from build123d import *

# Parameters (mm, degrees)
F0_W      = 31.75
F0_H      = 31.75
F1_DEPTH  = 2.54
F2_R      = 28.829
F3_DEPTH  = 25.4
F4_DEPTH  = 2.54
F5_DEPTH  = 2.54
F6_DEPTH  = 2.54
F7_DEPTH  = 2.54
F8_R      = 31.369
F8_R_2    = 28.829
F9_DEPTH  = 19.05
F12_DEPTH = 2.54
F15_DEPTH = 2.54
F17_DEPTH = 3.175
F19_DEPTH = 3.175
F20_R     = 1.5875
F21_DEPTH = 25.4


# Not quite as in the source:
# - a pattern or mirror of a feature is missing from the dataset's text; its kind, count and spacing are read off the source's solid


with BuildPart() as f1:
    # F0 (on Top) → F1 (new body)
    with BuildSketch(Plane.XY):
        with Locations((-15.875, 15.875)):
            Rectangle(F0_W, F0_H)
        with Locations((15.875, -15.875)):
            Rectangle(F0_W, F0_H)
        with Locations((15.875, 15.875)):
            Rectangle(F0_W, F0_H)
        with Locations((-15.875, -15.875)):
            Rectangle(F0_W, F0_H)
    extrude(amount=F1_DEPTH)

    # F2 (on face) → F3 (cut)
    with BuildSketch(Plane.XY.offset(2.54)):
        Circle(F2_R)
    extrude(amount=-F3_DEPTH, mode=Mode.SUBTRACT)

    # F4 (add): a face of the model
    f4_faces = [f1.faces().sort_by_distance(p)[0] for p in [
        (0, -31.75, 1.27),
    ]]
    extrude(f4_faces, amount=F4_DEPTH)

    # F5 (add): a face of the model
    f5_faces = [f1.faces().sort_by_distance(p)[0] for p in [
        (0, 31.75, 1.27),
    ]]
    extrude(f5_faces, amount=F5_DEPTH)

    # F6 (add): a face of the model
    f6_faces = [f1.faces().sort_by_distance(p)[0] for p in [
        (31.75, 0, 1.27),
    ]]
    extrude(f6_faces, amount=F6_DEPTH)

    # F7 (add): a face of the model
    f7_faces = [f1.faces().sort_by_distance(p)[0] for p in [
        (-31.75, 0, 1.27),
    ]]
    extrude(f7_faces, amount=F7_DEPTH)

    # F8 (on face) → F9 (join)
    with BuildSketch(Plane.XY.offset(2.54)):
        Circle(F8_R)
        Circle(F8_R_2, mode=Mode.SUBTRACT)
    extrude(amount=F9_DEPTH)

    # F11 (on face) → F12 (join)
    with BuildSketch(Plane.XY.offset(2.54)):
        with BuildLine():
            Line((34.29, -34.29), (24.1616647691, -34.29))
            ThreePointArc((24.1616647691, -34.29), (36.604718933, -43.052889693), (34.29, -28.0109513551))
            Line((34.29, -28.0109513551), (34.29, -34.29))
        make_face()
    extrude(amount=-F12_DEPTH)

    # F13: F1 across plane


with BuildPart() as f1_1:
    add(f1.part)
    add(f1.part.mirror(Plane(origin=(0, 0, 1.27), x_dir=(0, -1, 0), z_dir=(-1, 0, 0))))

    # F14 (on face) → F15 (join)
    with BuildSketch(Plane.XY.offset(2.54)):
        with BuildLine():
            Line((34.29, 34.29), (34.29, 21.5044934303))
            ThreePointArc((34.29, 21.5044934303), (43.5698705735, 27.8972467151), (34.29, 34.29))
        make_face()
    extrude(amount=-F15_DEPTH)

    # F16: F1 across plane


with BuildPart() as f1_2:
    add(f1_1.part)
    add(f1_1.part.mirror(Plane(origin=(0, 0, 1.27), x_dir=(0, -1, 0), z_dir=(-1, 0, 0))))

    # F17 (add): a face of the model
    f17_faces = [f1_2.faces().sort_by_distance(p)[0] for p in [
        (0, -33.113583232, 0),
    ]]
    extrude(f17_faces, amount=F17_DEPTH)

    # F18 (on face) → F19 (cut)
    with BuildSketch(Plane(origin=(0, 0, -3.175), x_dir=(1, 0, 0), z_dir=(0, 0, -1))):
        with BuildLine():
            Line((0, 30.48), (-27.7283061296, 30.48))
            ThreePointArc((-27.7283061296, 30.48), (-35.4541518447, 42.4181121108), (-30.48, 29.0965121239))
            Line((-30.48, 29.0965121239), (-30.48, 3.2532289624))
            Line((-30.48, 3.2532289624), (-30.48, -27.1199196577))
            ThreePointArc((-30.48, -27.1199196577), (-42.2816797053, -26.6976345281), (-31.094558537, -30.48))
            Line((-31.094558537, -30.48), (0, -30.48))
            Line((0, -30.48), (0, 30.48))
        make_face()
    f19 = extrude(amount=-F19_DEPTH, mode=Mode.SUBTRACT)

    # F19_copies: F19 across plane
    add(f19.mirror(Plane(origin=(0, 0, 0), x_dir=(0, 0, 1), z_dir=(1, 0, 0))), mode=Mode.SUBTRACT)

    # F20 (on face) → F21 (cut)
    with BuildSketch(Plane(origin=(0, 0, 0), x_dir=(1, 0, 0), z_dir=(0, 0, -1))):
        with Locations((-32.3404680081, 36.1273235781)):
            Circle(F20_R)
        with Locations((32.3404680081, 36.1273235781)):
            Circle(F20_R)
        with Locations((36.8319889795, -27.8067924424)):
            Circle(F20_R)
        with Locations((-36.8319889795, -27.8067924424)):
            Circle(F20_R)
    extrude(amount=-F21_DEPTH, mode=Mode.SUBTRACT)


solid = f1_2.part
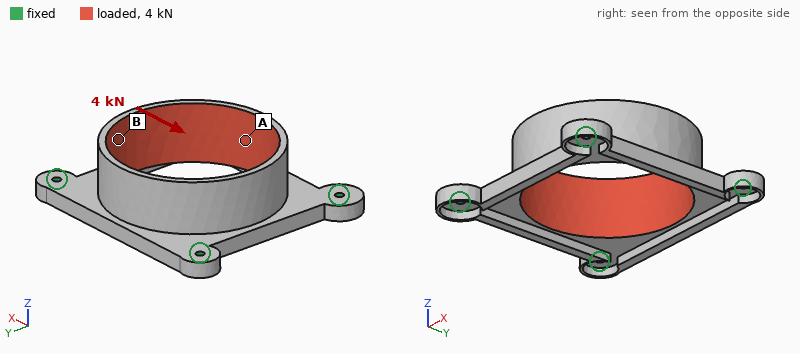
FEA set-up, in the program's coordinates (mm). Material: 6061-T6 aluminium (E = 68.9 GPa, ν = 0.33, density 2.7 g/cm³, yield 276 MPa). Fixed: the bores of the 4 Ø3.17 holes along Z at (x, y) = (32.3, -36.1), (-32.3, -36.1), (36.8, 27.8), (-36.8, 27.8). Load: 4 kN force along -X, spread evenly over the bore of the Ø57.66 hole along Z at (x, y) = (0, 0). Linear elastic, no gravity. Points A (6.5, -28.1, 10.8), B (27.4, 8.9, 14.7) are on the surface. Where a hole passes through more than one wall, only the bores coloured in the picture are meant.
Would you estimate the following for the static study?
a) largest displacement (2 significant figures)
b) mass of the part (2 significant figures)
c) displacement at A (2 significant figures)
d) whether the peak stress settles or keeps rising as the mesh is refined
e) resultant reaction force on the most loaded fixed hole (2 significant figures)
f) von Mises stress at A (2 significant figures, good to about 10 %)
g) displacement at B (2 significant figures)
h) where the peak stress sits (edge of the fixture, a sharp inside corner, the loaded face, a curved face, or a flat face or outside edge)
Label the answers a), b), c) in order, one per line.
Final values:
a) 0.13 mm
b) 51 g
c) 0.049 mm
d) keeps rising
e) 1.1 kN
f) 23 MPa
g) 0.091 mm
h) edge of the fixture
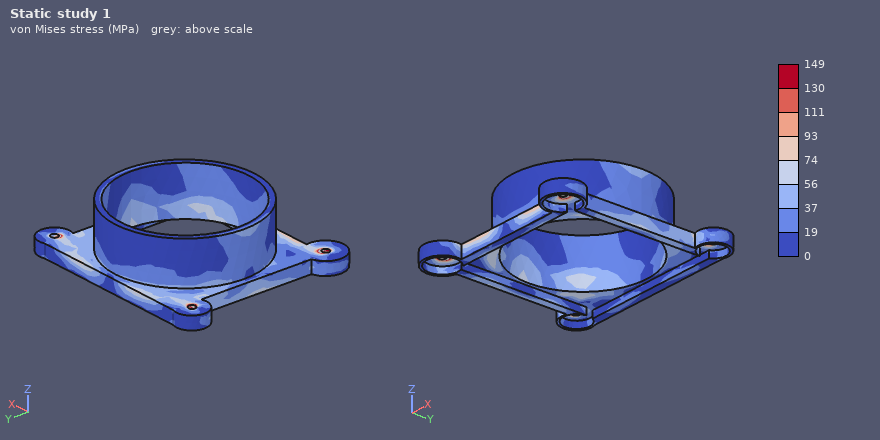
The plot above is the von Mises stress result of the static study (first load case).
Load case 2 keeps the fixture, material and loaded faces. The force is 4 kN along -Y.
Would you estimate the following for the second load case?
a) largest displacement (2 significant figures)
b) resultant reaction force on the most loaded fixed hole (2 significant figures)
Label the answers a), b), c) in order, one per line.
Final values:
a) 0.18 mm
b) 1.3 kN
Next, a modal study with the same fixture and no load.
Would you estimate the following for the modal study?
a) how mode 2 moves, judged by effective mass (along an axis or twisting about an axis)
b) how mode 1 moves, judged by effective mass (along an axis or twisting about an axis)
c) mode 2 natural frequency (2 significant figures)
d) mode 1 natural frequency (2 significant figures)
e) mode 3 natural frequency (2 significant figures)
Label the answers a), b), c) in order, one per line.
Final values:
a) along Z
b) along Z
c) 3700 Hz
d) 3400 Hz
e) 4100 Hz
